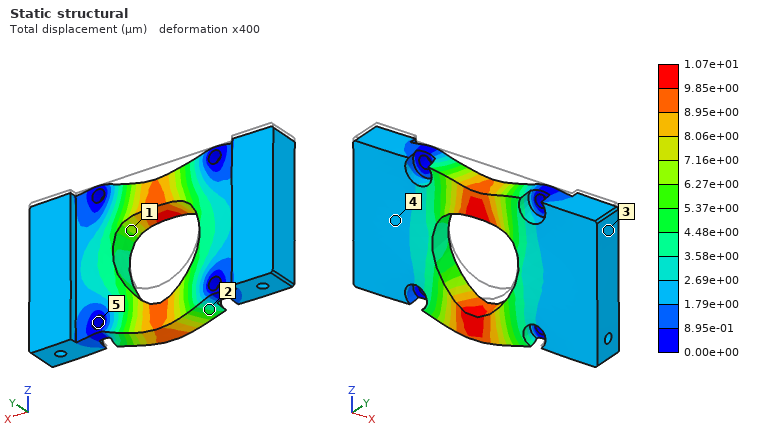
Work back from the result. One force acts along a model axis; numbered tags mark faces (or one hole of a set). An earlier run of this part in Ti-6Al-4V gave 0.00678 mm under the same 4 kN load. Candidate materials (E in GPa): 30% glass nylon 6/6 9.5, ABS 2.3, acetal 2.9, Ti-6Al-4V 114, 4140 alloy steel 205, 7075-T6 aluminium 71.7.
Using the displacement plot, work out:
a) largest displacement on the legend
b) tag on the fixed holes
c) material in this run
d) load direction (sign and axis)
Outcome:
1.07e+01 µm
5
7075-T6 aluminium
-Z
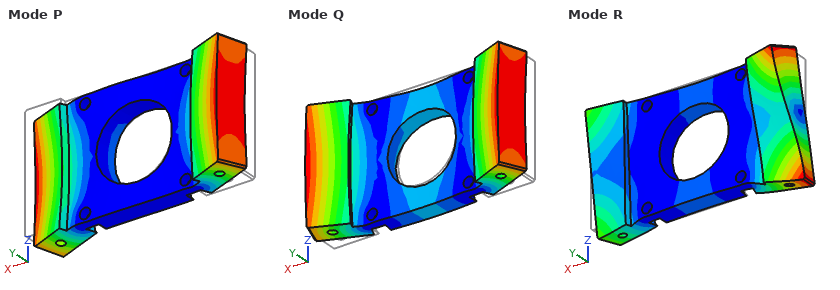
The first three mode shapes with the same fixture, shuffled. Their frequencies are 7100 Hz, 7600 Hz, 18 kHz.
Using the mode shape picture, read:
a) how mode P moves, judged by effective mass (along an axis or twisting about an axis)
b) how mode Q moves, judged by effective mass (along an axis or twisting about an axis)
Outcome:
twisting about Z
along Y
